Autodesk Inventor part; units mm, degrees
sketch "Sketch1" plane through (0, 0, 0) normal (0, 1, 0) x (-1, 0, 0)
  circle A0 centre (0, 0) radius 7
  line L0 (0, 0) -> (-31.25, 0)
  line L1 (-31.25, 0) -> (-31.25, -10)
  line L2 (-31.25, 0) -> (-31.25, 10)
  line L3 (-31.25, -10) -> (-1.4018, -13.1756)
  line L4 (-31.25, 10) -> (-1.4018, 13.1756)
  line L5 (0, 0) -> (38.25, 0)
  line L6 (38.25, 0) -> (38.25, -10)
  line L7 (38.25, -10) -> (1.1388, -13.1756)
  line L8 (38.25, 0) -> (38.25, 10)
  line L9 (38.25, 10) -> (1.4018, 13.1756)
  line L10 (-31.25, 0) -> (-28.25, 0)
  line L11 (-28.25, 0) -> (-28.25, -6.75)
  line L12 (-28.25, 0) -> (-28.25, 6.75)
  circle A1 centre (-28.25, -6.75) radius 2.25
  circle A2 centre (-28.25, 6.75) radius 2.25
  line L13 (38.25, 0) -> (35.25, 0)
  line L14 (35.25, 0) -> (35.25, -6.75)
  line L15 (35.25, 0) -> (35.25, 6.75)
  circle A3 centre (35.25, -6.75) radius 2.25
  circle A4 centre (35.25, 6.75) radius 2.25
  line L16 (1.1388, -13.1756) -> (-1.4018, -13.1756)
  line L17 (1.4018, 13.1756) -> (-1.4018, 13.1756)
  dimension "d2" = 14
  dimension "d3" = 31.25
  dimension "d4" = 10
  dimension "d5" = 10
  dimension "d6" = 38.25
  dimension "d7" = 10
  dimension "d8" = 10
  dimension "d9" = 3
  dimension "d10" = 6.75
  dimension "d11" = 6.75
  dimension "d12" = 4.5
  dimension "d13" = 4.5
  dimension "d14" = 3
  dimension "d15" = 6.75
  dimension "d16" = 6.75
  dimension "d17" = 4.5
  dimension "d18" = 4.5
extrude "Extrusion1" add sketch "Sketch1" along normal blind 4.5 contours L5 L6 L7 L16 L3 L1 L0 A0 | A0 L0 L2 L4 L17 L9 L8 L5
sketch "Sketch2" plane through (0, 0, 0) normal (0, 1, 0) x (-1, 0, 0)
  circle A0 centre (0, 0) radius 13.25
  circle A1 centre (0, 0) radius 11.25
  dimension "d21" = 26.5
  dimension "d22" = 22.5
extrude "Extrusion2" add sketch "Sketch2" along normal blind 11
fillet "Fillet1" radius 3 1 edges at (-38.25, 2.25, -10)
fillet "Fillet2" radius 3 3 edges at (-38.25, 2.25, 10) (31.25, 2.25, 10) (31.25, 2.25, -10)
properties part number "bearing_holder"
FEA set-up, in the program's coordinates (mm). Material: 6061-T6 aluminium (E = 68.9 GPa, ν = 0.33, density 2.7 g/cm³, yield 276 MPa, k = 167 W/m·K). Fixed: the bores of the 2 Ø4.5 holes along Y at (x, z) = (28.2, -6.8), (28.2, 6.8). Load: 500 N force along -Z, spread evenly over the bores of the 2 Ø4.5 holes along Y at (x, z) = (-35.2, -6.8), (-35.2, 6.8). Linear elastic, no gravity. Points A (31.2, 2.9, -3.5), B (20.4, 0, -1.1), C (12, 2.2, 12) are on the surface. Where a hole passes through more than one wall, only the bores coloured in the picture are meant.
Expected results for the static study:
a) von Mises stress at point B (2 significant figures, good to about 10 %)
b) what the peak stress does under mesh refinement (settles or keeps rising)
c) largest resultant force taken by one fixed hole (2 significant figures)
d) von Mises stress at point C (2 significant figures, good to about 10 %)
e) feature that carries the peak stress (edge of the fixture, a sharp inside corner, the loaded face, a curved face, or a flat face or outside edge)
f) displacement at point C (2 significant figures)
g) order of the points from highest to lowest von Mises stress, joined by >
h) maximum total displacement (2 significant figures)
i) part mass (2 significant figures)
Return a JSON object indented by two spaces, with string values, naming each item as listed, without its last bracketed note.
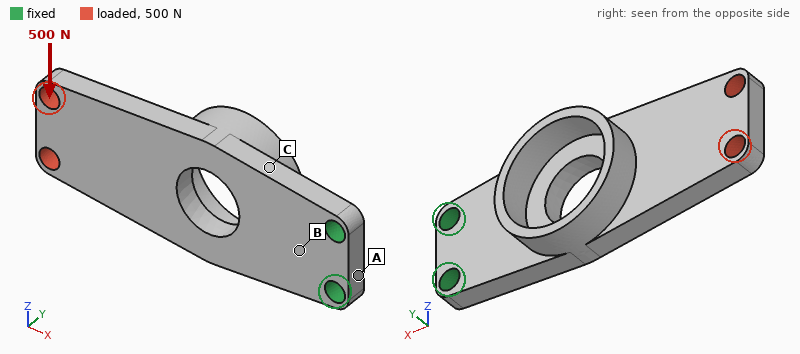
{
  "von Mises stress at point B": "24 MPa",
  "what the peak stress does under mesh refinement": "keeps rising",
  "largest resultant force taken by one fixed hole": "2.1 kN",
  "von Mises stress at point C": "69 MPa",
  "feature that carries the peak stress": "edge of the fixture",
  "displacement at point C": "0.026 mm",
  "order of the points from highest to lowest von Mises stress, joined by >": "C > B > A",
  "maximum total displacement": "0.17 mm",
  "part mass": "20 g"
}
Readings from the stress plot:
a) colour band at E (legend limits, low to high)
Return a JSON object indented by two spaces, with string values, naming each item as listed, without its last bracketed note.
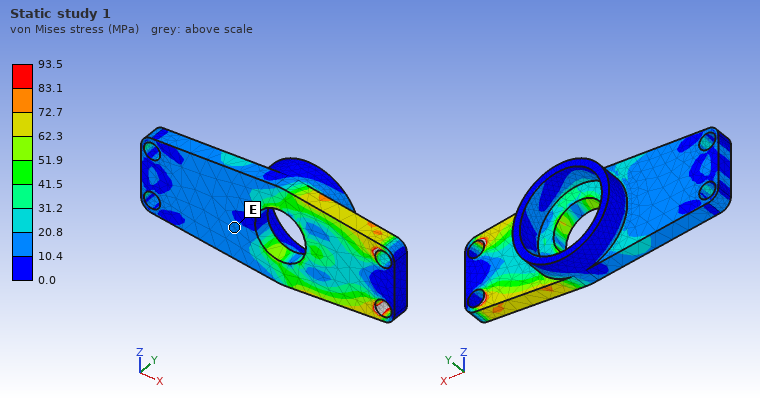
{
  "colour band at E": "10.4 to 20.8 MPa"
}
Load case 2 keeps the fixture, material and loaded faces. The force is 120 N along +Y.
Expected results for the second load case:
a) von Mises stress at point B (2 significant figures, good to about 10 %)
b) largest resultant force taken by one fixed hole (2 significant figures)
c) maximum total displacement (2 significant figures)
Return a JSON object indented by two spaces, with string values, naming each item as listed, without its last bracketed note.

{
  "von Mises stress at point B": "78 MPa",
  "largest resultant force taken by one fixed hole": "60 N",
  "maximum total displacement": "0.79 mm"
}
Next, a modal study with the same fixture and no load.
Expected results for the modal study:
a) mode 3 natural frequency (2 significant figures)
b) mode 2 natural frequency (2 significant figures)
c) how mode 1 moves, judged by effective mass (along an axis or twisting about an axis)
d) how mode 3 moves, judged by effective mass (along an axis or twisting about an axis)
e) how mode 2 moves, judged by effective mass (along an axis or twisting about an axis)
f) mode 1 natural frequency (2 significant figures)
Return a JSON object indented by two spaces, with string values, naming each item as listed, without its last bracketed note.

{
  "mode 3 natural frequency": "4600 Hz",
  "mode 2 natural frequency": "3700 Hz",
  "how mode 1 moves, judged by effective mass": "along Y",
  "how mode 3 moves, judged by effective mass": "twisting about X",
  "how mode 2 moves, judged by effective mass": "along Z",
  "mode 1 natural frequency": "930 Hz"
}
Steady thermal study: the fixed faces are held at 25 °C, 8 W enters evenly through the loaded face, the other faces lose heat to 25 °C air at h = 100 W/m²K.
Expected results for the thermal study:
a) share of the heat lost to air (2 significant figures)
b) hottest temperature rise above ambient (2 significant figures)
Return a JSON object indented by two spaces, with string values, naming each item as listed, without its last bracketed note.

{
  "share of the heat lost to air": "51 %",
  "hottest temperature rise above ambient": "23 K"
}
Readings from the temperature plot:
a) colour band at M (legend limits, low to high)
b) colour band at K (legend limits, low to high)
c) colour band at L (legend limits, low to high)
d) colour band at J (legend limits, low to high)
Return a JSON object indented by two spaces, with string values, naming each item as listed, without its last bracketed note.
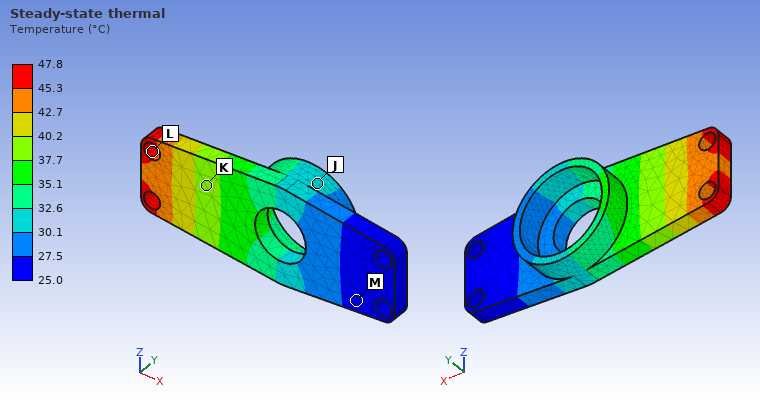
{
  "colour band at M": "25.0 to 27.5 °C",
  "colour band at K": "37.7 to 40.2 °C",
  "colour band at L": "45.3 to 47.8 °C",
  "colour band at J": "30.1 to 32.6 °C"
}
